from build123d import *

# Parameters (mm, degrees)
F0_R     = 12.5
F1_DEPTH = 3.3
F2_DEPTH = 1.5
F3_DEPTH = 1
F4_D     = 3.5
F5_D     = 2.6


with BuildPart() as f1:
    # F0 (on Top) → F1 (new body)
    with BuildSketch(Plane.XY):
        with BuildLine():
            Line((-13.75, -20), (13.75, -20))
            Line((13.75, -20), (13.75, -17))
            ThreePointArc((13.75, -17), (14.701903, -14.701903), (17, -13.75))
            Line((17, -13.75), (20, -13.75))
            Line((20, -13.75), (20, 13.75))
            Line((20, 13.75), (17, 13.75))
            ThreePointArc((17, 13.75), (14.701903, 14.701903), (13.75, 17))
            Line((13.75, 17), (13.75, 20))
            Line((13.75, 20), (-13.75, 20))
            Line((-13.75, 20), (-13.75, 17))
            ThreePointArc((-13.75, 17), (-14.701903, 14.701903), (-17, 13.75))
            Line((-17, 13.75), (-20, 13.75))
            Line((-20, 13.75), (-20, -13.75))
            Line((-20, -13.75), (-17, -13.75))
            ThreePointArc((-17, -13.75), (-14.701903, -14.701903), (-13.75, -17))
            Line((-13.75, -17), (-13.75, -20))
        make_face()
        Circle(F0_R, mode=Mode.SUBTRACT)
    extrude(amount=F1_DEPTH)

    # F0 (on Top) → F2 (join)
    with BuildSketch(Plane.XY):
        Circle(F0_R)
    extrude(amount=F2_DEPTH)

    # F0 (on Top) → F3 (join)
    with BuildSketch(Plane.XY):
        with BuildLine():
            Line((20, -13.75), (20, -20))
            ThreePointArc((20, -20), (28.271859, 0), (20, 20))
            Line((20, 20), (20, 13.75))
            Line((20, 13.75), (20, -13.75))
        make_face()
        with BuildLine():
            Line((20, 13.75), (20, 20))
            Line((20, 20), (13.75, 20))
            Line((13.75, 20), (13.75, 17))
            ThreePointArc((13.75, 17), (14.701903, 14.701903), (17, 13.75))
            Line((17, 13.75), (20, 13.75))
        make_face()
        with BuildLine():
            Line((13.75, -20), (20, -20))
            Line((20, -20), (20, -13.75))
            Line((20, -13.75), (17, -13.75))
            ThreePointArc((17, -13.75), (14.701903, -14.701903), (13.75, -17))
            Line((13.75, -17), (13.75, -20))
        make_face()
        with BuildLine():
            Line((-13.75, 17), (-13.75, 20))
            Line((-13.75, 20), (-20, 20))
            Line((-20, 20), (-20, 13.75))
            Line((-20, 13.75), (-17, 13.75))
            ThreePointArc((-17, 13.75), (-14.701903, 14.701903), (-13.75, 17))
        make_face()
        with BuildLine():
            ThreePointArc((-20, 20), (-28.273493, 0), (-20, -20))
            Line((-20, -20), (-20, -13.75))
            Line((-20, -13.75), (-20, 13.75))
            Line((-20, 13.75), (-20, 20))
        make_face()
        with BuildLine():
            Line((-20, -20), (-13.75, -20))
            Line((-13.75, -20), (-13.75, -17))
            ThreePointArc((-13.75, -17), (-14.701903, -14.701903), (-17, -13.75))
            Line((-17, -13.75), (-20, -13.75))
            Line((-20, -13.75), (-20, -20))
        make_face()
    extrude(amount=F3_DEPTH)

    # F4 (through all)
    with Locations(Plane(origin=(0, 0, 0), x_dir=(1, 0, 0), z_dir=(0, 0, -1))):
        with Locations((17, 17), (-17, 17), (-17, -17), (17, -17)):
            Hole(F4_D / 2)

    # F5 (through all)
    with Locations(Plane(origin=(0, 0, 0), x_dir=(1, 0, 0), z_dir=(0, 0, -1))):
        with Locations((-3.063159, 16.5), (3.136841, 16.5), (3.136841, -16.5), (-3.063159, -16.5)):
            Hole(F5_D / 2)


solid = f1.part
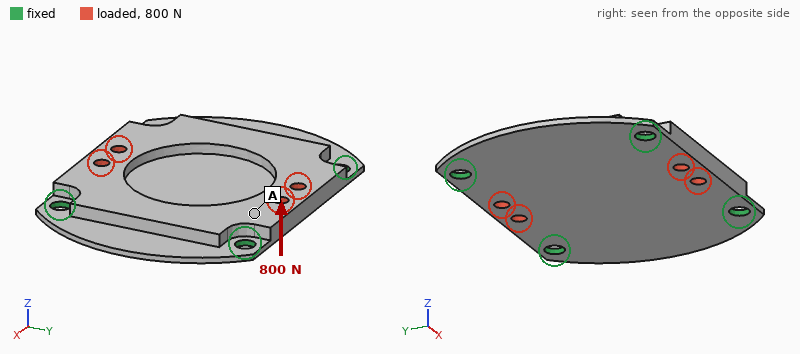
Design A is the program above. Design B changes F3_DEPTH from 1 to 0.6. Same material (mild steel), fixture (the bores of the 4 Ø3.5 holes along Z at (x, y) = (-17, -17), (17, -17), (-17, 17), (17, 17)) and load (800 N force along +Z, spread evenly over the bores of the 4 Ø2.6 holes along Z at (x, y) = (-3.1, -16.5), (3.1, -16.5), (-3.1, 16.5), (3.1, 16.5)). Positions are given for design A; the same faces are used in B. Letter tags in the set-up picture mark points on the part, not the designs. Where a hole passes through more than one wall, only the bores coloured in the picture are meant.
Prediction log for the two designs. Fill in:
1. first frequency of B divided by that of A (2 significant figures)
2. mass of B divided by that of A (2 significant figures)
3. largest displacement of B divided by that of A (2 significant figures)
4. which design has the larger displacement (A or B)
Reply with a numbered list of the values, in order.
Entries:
1. 0.92
2. 0.95
3. 1.2
4. B
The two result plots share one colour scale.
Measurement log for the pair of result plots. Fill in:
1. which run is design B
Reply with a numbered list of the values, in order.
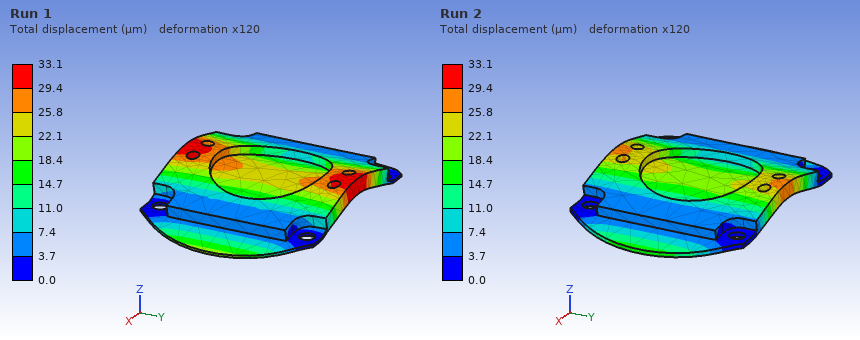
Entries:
1. Run 1
